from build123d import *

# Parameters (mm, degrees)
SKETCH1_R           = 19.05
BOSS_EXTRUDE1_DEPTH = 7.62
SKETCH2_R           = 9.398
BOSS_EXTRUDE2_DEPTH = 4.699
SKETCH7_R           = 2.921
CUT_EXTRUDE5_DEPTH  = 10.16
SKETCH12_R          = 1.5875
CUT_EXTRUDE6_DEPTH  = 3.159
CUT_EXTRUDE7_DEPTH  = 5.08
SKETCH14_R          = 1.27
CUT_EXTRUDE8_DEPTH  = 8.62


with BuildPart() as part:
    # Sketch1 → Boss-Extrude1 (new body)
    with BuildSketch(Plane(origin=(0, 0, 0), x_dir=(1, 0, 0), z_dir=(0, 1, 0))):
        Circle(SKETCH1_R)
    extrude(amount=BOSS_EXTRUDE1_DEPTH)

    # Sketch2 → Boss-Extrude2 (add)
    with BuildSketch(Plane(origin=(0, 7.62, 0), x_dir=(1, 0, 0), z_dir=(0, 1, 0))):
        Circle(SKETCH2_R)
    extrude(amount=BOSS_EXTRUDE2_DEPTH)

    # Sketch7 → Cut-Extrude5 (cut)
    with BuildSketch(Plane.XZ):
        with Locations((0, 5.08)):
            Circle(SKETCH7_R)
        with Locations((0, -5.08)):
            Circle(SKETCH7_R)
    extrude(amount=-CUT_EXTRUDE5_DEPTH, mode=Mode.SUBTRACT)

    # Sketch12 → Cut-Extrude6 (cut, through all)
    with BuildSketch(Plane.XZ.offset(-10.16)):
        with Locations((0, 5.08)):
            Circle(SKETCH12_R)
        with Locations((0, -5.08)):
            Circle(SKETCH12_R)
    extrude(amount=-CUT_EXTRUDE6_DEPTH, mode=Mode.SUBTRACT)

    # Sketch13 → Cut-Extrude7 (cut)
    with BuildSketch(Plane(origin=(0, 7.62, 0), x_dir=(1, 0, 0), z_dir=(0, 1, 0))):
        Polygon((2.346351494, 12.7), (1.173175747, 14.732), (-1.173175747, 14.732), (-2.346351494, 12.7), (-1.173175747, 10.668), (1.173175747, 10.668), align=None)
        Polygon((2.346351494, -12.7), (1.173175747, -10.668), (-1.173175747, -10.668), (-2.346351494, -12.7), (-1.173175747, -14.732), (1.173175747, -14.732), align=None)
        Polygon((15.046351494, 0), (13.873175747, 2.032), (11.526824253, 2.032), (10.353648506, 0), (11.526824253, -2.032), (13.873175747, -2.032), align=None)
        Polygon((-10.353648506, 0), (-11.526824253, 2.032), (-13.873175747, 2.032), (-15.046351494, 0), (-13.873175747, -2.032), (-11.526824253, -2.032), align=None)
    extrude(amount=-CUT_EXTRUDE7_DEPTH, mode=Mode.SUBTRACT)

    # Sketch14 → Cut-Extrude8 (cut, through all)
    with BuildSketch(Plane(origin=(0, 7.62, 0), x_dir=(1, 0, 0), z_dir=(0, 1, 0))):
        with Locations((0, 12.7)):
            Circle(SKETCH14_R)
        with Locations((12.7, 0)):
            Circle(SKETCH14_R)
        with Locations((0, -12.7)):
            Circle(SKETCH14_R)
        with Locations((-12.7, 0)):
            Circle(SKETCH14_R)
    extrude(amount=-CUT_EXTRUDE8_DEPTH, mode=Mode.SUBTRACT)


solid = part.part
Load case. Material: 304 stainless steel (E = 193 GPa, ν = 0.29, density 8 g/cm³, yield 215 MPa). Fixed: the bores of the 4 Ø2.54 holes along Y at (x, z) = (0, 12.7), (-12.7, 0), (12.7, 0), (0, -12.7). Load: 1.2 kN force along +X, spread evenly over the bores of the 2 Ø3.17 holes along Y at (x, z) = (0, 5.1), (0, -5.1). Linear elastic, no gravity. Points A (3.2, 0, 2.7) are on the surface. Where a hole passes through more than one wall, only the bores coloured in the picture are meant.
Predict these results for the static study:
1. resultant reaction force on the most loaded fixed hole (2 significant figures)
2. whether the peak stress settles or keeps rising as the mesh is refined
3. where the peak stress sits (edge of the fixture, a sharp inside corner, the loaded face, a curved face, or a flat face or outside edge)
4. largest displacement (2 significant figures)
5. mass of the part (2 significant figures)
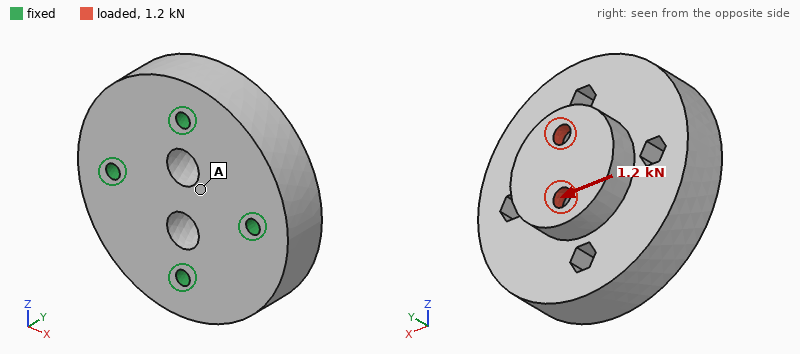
590 N
keeps rising
edge of the fixture
1.9 µm
73 g
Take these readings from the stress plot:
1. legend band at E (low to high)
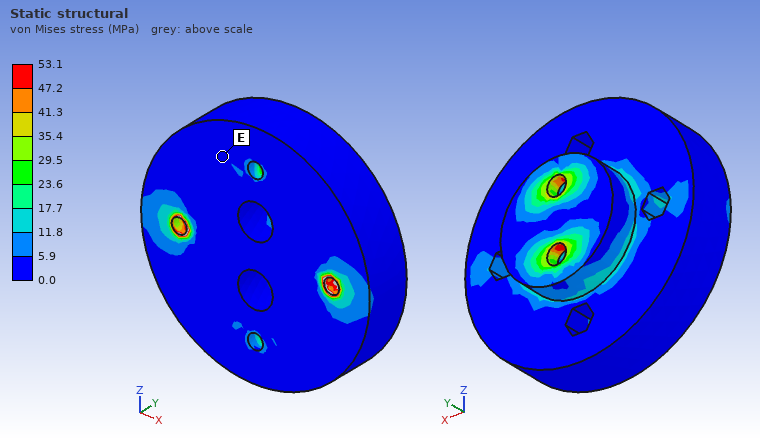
0.0 to 5.9 MPa
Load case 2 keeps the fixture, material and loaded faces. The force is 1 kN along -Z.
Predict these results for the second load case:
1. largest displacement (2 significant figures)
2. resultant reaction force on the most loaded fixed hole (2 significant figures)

2.1 µm
470 N
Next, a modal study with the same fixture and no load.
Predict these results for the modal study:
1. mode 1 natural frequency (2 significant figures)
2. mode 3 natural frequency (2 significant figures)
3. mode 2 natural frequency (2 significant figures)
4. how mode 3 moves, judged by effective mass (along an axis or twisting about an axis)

25 kHz
31 kHz
25 kHz
along Y
